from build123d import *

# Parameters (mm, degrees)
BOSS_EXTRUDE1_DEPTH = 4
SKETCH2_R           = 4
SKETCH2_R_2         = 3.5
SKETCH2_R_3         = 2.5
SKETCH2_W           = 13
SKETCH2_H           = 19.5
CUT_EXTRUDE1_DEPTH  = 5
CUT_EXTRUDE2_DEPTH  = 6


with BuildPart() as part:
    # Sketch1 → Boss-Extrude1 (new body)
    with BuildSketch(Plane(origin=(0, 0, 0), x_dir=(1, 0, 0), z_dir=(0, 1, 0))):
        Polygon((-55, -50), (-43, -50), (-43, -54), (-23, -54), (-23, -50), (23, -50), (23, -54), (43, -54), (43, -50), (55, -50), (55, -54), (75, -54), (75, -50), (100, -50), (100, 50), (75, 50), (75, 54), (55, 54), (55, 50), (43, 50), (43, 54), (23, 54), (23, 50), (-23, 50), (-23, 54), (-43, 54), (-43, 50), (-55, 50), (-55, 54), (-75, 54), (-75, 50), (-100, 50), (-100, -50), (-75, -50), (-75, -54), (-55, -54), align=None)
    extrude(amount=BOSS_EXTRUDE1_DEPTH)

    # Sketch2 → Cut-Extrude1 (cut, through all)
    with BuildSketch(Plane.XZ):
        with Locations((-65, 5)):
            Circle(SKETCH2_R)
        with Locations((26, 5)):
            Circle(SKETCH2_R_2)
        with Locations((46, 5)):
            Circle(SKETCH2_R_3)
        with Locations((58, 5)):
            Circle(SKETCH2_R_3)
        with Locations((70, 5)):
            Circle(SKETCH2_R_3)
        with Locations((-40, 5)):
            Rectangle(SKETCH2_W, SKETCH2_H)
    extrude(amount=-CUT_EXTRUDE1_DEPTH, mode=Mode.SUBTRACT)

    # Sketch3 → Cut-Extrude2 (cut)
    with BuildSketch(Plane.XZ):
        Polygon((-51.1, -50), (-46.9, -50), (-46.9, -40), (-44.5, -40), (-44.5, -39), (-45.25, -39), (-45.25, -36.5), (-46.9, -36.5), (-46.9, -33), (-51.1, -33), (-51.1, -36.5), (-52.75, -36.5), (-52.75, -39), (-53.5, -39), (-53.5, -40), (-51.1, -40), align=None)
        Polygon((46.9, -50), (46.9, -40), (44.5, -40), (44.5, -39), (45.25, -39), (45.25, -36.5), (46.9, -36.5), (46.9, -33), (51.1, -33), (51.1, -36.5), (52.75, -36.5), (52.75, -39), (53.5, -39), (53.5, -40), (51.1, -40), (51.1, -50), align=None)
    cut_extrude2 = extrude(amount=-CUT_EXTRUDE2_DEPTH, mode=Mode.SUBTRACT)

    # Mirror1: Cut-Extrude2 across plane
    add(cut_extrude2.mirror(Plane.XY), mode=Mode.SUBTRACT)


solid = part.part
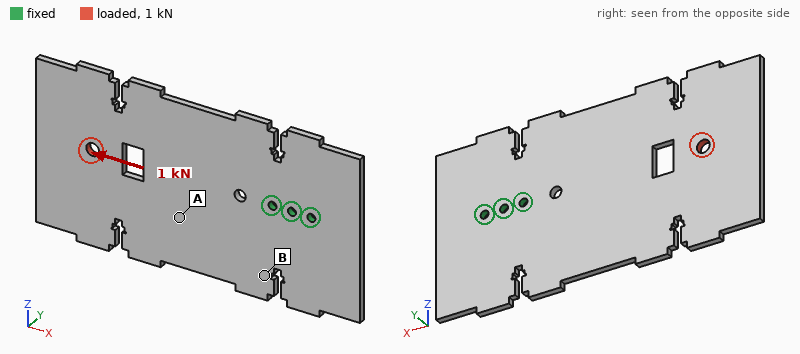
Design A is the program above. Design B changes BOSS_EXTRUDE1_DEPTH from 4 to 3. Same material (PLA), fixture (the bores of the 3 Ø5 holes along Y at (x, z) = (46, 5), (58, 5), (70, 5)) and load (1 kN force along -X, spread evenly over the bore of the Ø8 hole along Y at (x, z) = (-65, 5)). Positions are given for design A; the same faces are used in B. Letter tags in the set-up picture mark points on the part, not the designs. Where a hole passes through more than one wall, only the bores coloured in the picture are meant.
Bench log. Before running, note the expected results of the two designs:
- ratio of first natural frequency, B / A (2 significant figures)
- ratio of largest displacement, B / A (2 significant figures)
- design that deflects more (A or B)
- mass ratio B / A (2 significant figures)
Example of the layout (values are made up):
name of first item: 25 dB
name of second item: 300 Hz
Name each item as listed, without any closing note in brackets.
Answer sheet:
ratio of first natural frequency, B / A: 0.76
ratio of largest displacement, B / A: 1.3
design that deflects more: B
mass ratio B / A: 0.75
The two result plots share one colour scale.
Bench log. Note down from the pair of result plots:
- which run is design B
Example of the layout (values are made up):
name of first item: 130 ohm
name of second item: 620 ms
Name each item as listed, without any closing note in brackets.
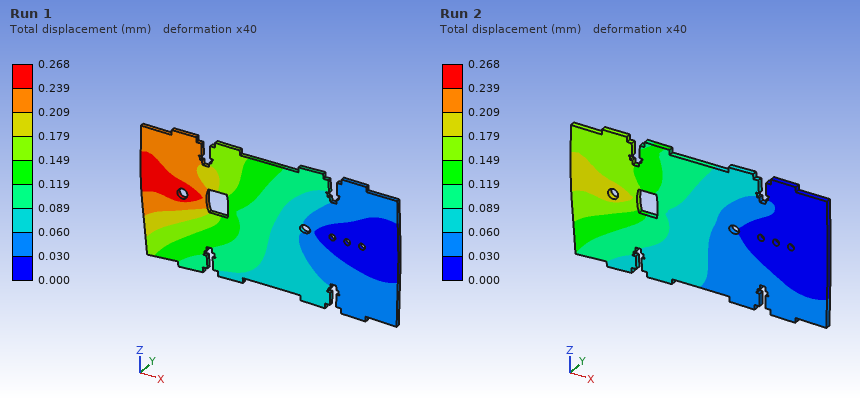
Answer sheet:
which run is design B: Run 1
